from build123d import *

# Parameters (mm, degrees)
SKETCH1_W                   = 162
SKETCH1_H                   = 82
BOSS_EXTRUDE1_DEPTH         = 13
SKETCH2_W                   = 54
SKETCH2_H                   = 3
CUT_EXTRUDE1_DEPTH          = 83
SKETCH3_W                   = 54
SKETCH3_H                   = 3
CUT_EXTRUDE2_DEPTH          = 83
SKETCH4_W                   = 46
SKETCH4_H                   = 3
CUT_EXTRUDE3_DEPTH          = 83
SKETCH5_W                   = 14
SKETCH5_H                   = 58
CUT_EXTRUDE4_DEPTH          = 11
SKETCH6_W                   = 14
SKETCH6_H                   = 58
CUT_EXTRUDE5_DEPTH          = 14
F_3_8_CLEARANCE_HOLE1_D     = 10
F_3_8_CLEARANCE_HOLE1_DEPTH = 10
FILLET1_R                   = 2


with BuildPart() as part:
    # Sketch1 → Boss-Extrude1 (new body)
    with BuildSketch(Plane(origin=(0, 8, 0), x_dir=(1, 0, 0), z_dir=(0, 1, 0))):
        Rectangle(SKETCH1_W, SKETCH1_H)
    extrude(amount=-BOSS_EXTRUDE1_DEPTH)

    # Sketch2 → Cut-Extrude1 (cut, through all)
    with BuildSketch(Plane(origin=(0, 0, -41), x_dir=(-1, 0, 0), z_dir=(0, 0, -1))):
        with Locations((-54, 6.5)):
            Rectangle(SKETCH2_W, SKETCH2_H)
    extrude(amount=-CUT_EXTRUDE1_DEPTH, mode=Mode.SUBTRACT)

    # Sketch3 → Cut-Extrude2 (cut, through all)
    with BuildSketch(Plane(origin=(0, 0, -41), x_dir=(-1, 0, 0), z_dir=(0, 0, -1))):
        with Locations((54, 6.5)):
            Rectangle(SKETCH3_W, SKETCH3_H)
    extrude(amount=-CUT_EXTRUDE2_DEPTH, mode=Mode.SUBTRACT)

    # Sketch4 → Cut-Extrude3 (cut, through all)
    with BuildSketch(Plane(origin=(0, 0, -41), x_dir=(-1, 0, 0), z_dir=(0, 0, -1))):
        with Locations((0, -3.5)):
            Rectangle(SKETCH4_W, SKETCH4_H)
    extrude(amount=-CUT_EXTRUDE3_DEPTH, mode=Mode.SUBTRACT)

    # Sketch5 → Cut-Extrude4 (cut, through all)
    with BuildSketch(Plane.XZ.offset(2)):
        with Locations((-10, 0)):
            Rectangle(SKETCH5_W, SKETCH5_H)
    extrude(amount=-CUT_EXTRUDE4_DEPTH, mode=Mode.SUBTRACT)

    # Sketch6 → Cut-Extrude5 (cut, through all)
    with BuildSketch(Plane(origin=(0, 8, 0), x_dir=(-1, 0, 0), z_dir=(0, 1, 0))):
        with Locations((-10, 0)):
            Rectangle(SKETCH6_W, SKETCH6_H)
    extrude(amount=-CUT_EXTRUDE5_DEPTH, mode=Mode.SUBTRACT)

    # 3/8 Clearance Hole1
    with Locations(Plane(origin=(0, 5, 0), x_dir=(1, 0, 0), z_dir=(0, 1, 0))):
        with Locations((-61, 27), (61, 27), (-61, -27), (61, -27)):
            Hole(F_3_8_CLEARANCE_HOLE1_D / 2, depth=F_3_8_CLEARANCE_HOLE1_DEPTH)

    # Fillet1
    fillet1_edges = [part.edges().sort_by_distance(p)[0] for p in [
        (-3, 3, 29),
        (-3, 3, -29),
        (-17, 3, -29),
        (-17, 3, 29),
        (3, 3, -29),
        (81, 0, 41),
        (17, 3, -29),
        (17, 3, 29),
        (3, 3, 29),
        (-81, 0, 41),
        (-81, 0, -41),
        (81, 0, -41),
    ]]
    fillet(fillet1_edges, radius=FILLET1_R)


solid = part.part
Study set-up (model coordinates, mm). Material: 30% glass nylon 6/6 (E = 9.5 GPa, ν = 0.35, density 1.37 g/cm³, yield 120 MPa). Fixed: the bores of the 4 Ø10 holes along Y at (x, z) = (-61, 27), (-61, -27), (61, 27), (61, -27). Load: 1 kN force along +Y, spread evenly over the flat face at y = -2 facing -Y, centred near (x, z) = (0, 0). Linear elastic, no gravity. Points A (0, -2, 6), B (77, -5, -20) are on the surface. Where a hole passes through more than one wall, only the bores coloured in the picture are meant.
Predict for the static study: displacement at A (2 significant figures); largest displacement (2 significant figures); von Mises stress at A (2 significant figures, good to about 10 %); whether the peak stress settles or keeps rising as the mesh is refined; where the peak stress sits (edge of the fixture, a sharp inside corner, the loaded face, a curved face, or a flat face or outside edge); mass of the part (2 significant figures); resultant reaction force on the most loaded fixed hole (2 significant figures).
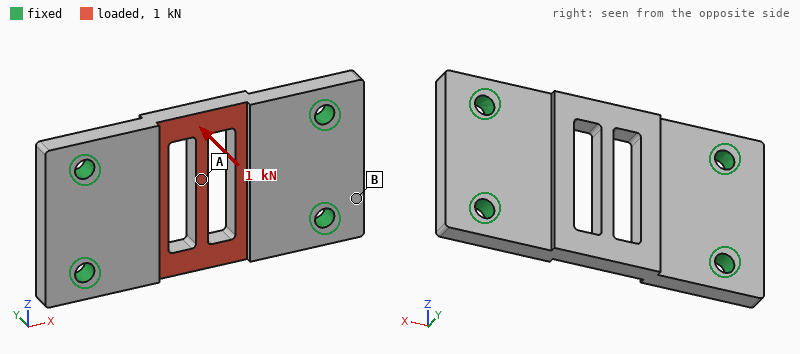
0.24 mm
0.24 mm
7.6 MPa
keeps rising
edge of the fixture
160 g
400 N
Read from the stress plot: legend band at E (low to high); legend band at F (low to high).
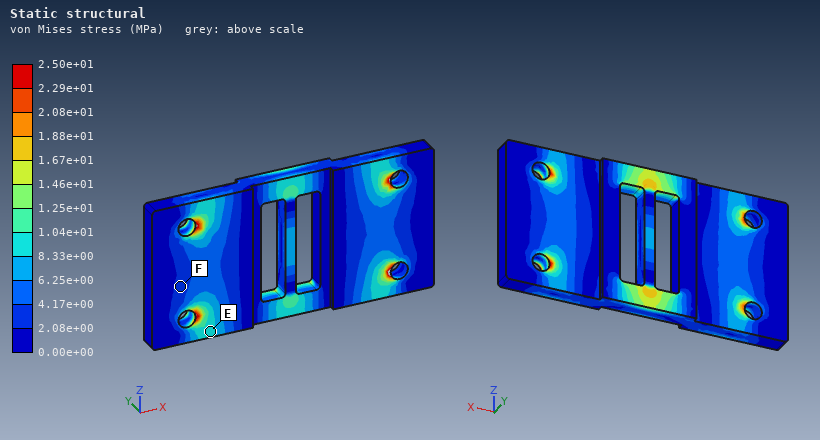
8.33e+00 to 1.04e+01 MPa
2.08e+00 to 4.17e+00 MPa
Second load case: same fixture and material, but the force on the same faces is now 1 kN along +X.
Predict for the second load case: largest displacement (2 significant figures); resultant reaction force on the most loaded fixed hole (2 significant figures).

96 µm
250 N
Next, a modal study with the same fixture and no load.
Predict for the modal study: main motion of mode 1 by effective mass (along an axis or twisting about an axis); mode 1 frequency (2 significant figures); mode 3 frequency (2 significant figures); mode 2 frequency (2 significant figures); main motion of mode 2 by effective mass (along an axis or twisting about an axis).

along Y
1900 Hz
3300 Hz
2600 Hz
twisting about X
